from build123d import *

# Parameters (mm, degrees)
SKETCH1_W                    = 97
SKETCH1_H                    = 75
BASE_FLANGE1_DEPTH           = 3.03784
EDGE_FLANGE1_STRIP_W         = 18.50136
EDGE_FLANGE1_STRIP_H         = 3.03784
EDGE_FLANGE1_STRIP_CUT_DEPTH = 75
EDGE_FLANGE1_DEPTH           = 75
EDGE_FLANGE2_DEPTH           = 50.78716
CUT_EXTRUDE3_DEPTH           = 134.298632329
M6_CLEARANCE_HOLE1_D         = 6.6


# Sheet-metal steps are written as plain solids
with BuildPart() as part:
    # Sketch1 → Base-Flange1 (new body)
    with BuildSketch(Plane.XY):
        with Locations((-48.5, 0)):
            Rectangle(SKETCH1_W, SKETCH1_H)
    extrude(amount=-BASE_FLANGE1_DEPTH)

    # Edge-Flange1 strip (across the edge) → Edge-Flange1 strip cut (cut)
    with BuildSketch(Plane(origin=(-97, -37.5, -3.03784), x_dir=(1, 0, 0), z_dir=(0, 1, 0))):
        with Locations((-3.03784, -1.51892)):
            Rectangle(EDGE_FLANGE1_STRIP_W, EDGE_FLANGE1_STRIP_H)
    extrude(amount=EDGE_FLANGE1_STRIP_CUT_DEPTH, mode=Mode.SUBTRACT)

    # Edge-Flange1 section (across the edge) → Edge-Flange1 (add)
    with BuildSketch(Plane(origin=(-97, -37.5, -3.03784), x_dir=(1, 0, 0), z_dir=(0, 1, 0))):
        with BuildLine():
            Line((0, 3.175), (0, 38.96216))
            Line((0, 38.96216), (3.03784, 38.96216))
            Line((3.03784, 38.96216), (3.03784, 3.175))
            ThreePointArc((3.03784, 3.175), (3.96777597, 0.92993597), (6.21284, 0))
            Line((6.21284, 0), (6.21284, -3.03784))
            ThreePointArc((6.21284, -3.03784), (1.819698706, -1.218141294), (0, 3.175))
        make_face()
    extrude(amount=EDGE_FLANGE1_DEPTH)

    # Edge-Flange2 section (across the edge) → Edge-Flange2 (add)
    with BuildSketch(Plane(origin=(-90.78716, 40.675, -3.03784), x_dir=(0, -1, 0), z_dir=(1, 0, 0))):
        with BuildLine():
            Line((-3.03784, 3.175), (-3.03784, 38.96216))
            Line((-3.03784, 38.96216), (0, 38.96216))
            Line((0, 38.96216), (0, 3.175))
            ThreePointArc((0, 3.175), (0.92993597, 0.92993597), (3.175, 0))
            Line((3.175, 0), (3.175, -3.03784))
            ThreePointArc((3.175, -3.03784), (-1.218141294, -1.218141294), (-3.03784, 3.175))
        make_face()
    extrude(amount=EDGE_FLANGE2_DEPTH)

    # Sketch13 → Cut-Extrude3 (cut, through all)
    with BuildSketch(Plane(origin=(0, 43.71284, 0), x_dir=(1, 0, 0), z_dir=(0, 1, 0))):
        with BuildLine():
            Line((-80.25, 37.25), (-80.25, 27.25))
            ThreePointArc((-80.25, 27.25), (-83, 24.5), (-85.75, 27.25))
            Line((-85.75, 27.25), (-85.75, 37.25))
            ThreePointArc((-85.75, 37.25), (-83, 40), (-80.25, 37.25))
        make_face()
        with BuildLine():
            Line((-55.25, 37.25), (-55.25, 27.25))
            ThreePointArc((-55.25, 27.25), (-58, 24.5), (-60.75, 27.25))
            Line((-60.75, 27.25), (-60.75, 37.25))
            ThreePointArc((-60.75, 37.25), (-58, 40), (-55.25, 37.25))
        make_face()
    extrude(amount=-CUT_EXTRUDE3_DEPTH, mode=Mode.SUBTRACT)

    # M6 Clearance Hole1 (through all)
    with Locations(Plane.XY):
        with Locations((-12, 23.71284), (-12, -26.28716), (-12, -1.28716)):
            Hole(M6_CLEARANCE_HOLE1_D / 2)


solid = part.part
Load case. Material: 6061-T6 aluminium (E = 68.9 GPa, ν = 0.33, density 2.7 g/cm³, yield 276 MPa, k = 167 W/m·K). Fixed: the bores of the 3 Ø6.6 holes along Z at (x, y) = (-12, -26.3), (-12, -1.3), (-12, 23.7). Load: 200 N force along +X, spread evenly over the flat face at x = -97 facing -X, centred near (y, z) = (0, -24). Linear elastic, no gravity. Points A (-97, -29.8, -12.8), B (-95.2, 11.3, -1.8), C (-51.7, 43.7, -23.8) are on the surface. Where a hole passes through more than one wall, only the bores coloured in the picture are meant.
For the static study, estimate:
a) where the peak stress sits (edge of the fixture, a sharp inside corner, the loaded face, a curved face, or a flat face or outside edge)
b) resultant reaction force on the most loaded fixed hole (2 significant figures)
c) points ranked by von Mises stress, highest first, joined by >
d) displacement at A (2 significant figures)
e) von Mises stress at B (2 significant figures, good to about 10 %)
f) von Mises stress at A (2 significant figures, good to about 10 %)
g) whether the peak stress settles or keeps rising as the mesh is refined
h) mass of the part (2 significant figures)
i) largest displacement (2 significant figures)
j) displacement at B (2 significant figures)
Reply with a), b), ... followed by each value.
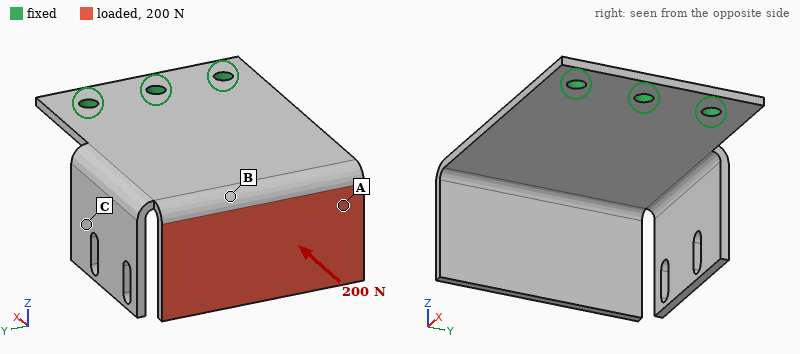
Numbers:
a) a sharp inside corner
b) 77 N
c) B > A > C
d) 1.1 mm
e) 28 MPa
f) 15 MPa
g) keeps rising
h) 98 g
i) 1.5 mm
j) 1.0 mm
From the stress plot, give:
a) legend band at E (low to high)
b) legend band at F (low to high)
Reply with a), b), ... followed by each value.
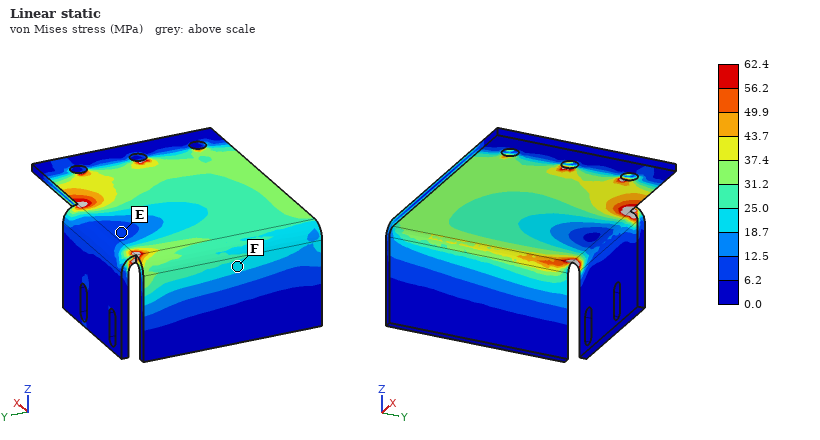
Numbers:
a) 6.2 to 12.5 MPa
b) 18.7 to 25.0 MPa
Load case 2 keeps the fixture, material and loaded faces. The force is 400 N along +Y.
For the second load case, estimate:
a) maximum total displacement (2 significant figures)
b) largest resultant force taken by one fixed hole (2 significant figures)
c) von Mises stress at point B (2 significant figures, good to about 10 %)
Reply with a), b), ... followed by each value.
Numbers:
a) 1.5 mm
b) 670 N
c) 29 MPa
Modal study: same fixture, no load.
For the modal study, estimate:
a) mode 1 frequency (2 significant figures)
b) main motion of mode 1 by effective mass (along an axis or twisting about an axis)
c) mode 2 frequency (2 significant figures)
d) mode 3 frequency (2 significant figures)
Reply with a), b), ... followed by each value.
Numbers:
a) 200 Hz
b) along Z
c) 420 Hz
d) 930 Hz
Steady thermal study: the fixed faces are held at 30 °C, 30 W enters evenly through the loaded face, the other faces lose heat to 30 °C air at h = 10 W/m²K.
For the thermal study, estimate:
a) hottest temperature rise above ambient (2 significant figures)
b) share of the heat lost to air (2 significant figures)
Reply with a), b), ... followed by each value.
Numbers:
a) 66 K
b) 23 %
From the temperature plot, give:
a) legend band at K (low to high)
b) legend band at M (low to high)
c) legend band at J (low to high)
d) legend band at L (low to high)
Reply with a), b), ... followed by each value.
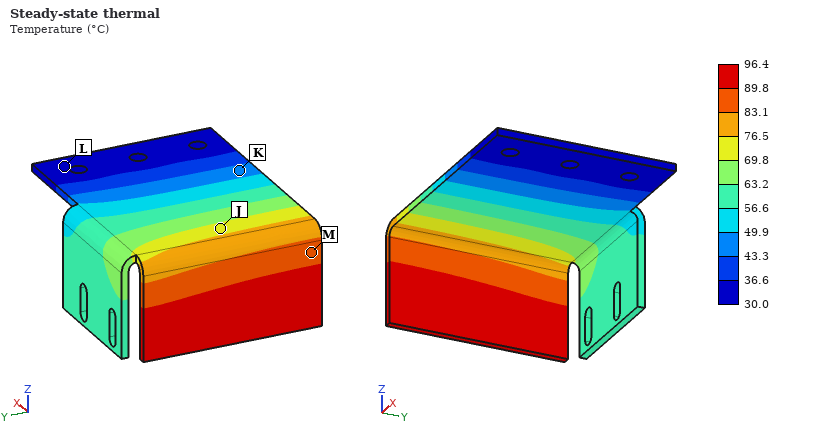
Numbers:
a) 43.3 to 49.9 °C
b) 83.1 to 89.8 °C
c) 69.8 to 76.5 °C
d) 30.0 to 36.6 °C
